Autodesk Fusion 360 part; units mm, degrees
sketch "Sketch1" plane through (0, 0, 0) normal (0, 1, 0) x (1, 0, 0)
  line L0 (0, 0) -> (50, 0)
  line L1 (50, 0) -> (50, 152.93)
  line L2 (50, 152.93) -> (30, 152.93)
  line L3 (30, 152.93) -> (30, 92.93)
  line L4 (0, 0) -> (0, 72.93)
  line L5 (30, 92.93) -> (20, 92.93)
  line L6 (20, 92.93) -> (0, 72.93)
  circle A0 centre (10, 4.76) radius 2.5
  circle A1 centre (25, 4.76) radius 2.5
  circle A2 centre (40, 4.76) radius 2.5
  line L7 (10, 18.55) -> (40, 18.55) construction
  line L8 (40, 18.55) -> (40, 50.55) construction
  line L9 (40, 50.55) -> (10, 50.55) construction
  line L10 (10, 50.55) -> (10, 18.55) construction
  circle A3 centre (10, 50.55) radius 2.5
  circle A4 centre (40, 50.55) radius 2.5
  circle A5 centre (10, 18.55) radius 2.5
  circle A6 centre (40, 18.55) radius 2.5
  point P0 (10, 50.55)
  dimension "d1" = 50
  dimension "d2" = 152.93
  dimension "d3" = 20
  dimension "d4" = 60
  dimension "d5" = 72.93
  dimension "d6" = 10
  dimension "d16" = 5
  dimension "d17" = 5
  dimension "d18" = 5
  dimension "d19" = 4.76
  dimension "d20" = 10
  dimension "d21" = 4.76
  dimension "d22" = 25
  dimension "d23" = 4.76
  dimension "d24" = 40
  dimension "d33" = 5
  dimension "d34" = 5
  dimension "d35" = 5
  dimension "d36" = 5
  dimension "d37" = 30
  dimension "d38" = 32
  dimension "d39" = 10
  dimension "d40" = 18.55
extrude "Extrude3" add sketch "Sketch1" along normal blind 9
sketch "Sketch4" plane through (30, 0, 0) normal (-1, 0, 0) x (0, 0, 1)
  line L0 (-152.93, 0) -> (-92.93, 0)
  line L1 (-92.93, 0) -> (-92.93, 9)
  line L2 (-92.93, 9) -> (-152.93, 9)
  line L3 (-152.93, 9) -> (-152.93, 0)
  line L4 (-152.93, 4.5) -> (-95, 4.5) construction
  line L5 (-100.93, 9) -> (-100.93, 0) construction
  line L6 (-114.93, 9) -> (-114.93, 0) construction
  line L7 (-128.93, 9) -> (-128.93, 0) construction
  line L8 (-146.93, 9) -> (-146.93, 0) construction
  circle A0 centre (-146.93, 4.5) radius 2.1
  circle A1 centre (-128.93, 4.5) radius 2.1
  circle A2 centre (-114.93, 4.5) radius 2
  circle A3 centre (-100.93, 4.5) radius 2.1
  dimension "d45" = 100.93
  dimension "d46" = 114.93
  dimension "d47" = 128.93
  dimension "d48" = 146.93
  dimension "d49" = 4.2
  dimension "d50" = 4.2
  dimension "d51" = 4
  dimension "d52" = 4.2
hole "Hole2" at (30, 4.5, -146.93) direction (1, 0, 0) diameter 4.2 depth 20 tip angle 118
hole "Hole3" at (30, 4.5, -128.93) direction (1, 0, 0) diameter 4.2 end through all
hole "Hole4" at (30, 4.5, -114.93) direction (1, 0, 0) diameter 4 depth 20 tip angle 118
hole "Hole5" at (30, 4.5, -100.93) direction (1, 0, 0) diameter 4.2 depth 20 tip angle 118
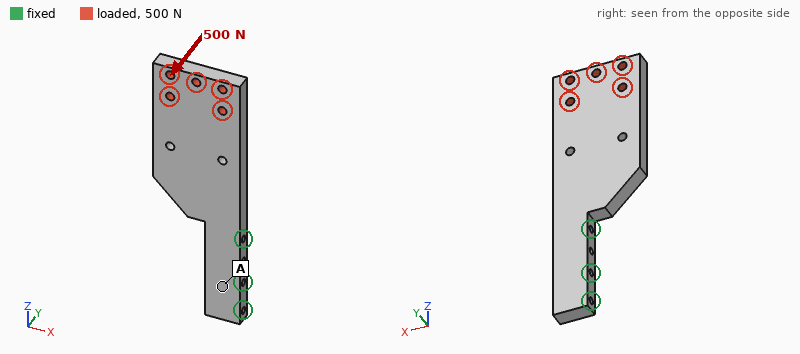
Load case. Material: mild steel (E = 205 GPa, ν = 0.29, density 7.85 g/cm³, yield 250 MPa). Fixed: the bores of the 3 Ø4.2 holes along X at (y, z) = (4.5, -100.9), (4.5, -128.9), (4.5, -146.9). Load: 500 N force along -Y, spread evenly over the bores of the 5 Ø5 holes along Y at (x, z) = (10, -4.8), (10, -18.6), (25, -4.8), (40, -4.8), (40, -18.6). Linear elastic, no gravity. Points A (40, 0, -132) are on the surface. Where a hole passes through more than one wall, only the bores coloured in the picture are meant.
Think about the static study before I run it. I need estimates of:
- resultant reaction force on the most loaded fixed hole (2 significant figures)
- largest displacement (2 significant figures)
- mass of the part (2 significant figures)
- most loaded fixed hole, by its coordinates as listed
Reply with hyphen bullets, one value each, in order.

- 800 N
- 0.46 mm
- 380 g
- (4.5, -100.9)
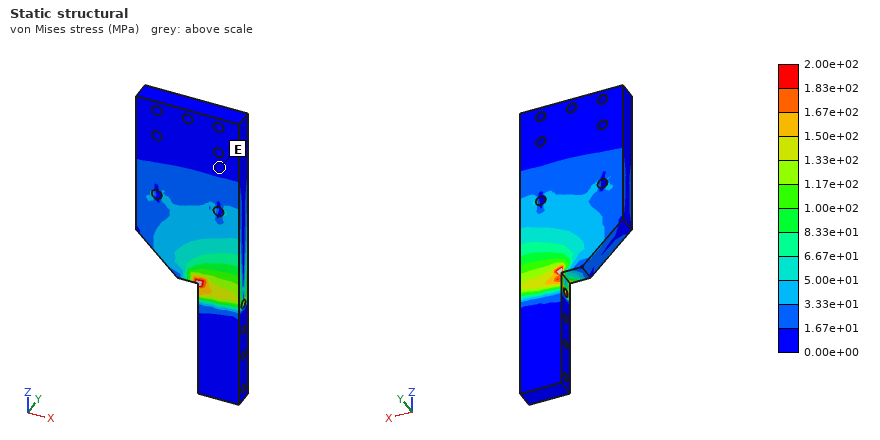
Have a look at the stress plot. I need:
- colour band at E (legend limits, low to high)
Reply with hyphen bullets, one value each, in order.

- 0.00e+00 to 1.67e+01 MPa
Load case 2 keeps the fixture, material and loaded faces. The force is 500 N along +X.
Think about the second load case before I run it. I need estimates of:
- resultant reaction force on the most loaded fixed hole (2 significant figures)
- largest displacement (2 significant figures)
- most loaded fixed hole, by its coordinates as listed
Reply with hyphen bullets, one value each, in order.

- 550 N
- 65 µm
- (4.5, -100.9)
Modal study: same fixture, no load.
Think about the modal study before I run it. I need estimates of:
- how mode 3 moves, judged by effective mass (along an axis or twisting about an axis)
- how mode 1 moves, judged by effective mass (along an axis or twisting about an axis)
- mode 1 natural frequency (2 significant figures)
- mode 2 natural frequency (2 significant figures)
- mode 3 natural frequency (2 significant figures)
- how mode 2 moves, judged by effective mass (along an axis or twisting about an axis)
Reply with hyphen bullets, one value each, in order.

- twisting about Z
- along Y
- 520 Hz
- 1300 Hz
- 2000 Hz
- along X
